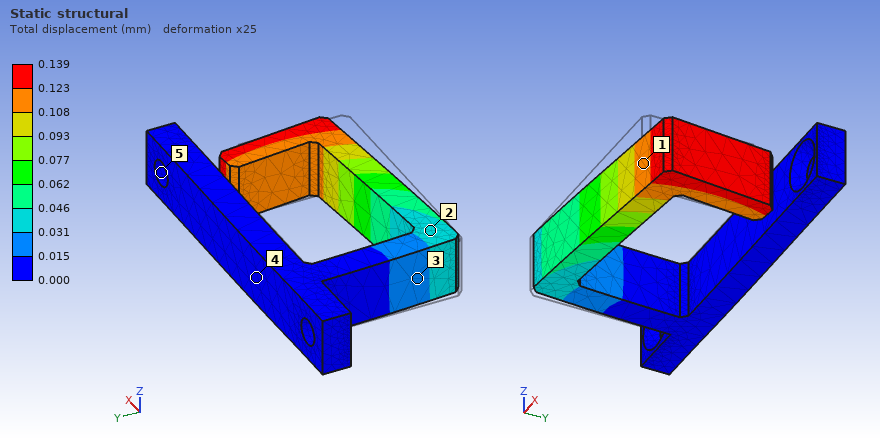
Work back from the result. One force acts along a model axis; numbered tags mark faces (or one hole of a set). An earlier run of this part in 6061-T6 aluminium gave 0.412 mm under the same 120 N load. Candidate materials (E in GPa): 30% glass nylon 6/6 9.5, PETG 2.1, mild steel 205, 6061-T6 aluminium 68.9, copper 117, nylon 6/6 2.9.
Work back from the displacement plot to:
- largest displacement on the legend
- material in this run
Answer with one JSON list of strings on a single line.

["0.139 mm", "mild steel"]
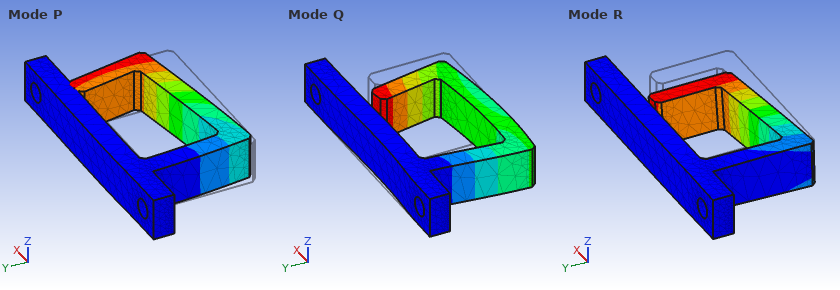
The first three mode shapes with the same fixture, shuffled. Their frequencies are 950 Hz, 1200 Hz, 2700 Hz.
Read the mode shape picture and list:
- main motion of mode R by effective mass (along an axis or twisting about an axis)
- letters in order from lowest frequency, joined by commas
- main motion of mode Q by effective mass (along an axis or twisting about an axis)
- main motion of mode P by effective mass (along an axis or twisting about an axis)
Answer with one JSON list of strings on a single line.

["along Z", "P, R, Q", "along X", "along Y"]
